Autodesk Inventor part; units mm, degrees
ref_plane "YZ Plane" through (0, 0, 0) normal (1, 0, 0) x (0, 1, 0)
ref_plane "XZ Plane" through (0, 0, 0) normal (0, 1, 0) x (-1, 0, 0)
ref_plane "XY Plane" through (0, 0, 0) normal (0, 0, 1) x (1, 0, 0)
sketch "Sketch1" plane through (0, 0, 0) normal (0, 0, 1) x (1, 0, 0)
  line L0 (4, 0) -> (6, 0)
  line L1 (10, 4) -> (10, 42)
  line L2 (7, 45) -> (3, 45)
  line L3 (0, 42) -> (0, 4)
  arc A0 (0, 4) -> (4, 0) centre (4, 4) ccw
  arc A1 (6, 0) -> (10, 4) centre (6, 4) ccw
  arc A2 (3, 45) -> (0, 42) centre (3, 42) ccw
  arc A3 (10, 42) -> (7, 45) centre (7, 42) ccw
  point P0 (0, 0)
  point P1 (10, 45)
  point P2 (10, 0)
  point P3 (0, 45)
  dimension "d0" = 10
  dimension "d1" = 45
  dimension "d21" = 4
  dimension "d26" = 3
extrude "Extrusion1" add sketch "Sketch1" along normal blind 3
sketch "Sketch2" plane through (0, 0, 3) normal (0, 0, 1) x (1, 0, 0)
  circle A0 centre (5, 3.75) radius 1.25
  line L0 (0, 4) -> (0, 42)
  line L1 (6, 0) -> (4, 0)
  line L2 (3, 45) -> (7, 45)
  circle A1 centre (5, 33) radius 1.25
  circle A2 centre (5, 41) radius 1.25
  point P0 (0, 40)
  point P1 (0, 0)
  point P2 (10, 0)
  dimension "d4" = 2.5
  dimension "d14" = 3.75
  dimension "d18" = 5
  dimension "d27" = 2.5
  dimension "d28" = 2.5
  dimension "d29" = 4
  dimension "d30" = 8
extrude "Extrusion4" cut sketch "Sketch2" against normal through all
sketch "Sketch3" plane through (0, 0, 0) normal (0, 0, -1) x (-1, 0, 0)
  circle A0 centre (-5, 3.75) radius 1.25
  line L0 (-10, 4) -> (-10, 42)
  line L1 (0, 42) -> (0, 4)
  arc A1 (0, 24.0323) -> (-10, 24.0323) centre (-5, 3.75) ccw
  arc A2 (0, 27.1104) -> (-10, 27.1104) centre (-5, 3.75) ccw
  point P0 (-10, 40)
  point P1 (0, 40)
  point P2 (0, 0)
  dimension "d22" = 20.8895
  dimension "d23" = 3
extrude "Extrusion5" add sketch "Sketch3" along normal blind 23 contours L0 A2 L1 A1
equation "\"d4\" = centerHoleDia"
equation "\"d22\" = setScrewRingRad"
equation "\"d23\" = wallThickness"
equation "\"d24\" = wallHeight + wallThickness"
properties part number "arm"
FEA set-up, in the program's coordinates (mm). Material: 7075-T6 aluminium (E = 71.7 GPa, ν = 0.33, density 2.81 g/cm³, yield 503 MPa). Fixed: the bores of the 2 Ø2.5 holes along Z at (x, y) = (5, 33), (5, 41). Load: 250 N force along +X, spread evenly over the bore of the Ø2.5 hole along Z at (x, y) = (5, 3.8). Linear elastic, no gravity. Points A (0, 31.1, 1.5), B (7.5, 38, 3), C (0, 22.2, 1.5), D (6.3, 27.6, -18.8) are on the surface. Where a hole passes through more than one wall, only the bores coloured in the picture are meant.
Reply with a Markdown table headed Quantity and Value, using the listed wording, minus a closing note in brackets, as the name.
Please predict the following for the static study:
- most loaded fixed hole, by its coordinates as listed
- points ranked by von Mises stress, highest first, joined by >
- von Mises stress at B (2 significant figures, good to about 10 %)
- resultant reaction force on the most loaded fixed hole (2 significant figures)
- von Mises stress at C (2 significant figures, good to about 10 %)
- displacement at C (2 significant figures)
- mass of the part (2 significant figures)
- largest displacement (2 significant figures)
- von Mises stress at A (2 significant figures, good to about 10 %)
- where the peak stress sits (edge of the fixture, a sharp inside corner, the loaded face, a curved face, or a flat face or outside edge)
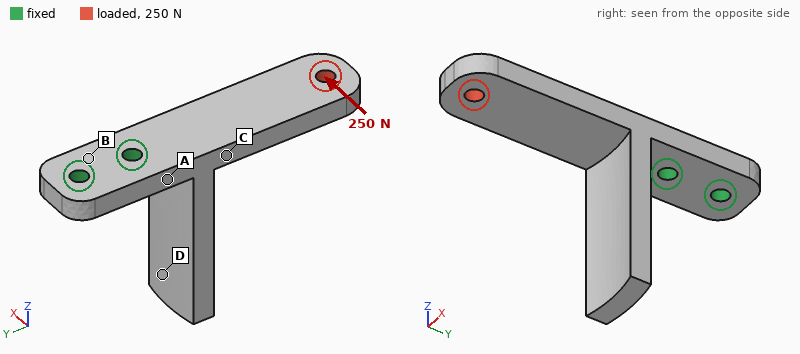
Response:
| Quantity | Value |
|---|---|
| most loaded fixed hole, by its coordinates as listed | (5, 33) |
| points ranked by von Mises stress, highest first, joined by > | A > C > B > D |
| von Mises stress at B | 47 MPa |
| resultant reaction force on the most loaded fixed hole | 780 N |
| von Mises stress at C | 92 MPa |
| displacement at C | 0.048 mm |
| mass of the part | 5.5 g |
| largest displacement | 0.20 mm |
| von Mises stress at A | 130 MPa |
| where the peak stress sits | edge of the fixture |
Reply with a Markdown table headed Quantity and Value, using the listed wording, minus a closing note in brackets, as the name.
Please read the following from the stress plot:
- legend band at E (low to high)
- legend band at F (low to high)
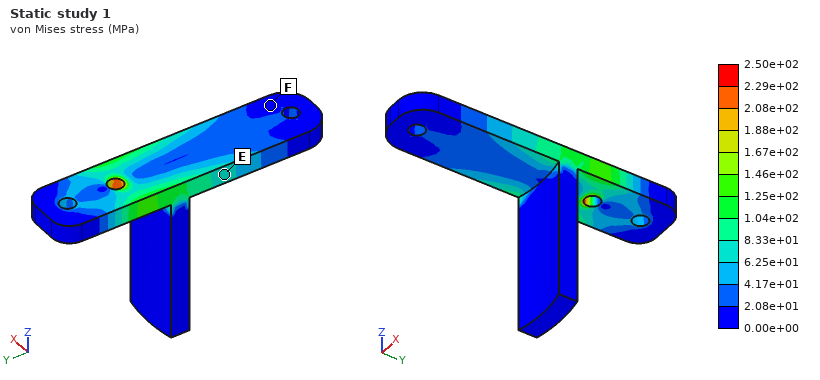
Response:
| Quantity | Value |
|---|---|
| legend band at E | 6.25e+01 to 8.33e+01 MPa |
| legend band at F | 0.00e+00 to 2.08e+01 MPa |
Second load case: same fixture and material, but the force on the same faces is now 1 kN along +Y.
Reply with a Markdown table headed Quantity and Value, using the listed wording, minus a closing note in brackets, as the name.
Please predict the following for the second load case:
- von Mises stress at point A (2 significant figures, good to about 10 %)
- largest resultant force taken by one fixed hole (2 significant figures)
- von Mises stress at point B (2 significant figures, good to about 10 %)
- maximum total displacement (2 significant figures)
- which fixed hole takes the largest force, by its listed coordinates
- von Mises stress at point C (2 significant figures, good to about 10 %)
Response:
| Quantity | Value |
|---|---|
| von Mises stress at point A | 18 MPa |
| largest resultant force taken by one fixed hole | 840 N |
| von Mises stress at point B | 8.2 MPa |
| maximum total displacement | 18 µm |
| which fixed hole takes the largest force, by its listed coordinates | (5, 33) |
| von Mises stress at point C | 33 MPa |
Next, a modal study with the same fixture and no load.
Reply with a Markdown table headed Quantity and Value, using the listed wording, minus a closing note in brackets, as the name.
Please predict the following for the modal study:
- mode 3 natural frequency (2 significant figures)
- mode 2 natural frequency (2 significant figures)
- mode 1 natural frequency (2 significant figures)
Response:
| Quantity | Value |
|---|---|
| mode 3 natural frequency | 4400 Hz |
| mode 2 natural frequency | 4300 Hz |
| mode 1 natural frequency | 2100 Hz |
